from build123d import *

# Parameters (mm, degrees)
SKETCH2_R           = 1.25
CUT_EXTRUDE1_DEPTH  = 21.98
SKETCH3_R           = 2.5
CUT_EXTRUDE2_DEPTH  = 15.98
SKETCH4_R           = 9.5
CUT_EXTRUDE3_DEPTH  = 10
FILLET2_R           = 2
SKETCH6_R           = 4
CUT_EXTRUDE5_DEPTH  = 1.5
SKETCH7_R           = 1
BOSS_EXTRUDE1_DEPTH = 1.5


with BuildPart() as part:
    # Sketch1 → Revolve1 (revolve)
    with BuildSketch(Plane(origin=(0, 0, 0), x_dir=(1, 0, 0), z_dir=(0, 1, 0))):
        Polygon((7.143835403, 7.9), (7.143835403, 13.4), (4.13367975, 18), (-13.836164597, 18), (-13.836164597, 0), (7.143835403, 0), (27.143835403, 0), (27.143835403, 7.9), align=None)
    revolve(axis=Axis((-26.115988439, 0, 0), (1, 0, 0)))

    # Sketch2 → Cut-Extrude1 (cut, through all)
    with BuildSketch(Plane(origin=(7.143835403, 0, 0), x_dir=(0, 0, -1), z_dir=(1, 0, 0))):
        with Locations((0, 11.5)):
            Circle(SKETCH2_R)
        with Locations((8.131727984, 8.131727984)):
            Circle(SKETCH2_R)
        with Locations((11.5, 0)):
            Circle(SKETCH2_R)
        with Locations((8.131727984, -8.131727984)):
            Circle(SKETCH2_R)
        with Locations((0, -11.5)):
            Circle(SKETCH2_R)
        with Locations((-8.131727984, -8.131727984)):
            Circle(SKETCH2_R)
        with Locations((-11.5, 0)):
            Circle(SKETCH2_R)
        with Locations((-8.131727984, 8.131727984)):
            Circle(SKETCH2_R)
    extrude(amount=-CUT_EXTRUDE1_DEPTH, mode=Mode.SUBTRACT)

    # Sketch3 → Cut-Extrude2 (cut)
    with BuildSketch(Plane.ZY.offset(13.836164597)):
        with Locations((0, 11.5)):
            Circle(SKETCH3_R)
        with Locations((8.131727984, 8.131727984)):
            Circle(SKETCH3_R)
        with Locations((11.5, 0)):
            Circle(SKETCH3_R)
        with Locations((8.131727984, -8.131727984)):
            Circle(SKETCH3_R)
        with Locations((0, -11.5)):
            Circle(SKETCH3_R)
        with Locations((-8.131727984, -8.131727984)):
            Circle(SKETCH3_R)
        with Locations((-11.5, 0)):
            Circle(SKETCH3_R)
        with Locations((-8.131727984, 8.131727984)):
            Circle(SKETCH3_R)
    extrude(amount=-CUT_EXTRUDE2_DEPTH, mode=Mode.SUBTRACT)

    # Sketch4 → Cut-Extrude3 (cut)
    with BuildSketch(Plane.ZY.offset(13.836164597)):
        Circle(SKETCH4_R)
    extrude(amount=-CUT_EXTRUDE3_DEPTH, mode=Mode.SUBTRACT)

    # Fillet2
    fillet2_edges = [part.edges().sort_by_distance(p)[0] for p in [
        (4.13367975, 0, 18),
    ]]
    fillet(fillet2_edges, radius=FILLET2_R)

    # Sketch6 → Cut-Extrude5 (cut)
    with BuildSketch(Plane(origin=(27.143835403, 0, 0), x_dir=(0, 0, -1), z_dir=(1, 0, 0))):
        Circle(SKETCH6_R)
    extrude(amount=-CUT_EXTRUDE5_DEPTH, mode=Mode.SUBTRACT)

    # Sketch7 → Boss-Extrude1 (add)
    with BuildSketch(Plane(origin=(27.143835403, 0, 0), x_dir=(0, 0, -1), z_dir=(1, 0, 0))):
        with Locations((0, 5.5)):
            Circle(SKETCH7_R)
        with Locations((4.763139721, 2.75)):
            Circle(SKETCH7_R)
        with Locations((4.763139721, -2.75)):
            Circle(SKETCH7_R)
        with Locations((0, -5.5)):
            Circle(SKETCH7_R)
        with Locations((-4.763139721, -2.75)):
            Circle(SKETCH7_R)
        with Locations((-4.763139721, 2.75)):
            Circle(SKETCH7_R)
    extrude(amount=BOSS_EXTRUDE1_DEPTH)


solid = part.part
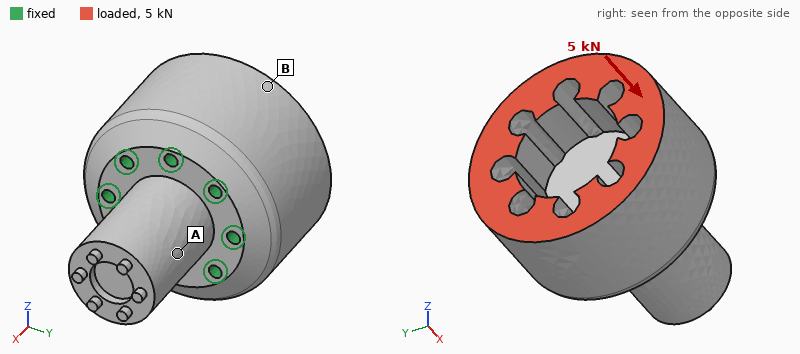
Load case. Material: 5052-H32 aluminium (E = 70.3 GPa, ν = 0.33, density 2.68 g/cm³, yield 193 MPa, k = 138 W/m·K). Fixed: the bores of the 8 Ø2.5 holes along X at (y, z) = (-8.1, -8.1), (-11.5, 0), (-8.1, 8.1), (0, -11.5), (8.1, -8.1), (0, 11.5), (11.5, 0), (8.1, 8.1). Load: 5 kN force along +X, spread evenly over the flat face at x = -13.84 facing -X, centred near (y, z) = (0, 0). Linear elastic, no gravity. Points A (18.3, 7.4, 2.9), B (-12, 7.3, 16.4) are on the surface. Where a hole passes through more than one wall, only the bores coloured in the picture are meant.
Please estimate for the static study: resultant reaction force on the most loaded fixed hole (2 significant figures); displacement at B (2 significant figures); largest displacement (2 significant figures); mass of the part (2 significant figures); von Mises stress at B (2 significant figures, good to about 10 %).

630 N
3.7 µm
4.0 µm
51 g
9.9 MPa
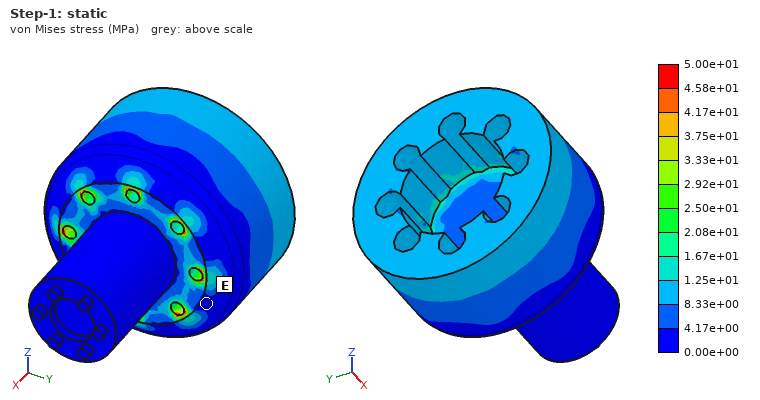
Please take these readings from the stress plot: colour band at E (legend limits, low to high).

0.00e+00 to 4.17e+00 MPa
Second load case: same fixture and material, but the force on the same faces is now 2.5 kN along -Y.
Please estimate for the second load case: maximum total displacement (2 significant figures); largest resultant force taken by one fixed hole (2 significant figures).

15 µm
850 N
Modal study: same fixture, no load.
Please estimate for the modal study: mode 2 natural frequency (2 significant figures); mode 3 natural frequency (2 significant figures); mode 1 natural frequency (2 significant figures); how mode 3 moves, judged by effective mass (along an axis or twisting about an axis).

18 kHz
23 kHz
18 kHz
along Z
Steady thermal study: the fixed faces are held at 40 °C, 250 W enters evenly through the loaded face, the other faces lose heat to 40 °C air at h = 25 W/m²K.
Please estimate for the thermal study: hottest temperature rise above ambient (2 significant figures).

60 K
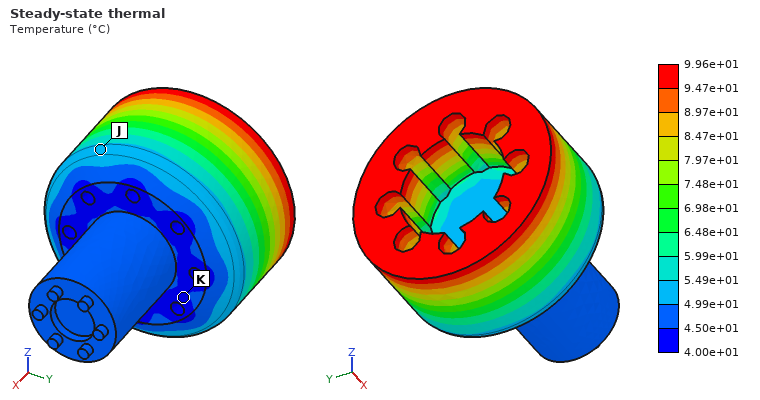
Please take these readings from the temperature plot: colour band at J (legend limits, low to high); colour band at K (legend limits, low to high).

4.99e+01 to 5.49e+01 °C
4.00e+01 to 4.50e+01 °C
